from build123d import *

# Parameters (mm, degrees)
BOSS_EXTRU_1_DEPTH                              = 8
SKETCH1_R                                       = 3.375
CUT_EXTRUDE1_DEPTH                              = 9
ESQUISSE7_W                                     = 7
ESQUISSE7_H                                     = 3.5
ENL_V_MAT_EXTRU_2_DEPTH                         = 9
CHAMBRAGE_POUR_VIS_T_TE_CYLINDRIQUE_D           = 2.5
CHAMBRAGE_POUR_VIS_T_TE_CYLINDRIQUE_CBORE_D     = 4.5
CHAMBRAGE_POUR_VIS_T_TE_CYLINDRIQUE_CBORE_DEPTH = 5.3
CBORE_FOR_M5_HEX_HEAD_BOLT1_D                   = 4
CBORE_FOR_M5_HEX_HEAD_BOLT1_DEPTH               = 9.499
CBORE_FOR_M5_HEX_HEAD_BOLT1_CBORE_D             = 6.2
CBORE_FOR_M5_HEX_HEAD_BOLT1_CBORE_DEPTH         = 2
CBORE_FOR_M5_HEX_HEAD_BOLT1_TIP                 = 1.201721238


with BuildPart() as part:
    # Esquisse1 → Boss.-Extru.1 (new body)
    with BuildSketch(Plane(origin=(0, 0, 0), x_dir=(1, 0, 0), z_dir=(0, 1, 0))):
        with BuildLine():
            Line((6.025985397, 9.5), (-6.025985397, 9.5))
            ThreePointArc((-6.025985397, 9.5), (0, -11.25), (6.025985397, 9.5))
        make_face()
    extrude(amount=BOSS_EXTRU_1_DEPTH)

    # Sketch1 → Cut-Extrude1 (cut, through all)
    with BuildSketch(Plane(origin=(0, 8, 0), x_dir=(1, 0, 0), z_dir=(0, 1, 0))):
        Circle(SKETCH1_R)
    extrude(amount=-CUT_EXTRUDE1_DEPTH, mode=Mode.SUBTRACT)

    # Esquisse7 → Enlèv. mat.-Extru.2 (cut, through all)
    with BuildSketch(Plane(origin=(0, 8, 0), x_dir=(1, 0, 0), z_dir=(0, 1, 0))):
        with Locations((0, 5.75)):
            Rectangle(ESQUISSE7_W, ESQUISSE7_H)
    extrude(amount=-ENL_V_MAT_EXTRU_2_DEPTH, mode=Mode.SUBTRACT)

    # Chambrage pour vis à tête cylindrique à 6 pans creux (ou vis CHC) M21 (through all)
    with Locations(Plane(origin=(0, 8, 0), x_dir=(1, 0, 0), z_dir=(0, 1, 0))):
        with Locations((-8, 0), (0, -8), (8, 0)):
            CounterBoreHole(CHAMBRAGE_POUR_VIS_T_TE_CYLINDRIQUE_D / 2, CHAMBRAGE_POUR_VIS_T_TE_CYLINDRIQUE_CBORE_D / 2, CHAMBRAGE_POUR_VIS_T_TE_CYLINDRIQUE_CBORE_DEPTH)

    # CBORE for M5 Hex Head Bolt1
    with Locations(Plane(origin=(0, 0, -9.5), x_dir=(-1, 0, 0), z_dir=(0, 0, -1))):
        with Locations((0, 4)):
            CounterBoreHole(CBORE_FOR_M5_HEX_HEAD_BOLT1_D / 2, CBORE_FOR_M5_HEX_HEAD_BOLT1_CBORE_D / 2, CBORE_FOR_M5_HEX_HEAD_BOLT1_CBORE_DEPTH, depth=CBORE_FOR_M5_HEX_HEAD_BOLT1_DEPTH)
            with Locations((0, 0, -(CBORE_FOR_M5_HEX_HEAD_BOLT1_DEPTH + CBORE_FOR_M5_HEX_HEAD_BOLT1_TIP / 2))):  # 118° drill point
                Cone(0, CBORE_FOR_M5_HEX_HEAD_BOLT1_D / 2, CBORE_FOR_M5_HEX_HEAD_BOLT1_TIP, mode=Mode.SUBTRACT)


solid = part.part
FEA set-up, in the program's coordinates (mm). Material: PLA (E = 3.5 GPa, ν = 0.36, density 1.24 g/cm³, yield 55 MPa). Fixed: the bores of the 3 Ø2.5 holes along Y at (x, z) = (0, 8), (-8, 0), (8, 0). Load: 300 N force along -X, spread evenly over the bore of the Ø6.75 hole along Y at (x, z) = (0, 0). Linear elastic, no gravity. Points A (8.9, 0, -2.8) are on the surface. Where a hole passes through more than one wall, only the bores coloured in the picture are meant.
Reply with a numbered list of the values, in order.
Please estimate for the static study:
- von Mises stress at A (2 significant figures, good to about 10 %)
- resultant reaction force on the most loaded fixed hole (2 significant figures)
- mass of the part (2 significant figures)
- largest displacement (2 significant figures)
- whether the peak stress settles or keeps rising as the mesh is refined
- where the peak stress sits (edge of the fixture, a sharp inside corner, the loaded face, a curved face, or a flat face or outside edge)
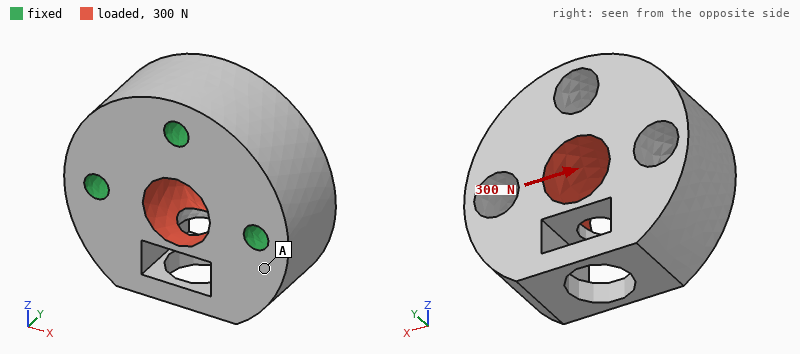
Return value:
1. 1.9 MPa
2. 130 N
3. 2.8 g
4. 21 µm
5. keeps rising
6. edge of the fixture
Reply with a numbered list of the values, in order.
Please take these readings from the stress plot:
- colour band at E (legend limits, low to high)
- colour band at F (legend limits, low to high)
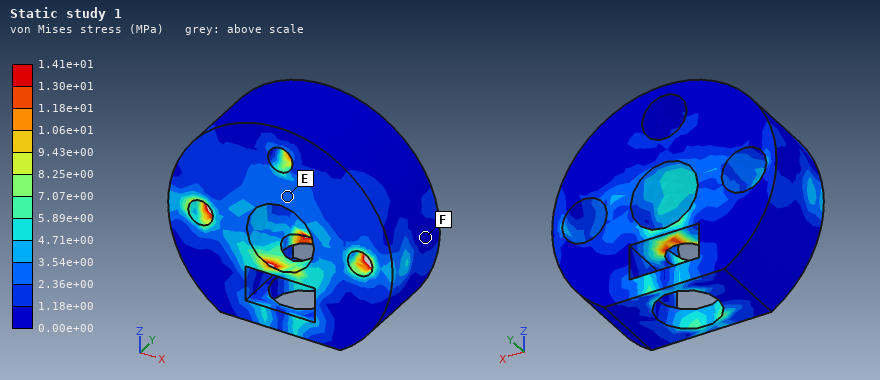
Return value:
1. 2.36e+00 to 3.54e+00 MPa
2. 0.00e+00 to 1.18e+00 MPa
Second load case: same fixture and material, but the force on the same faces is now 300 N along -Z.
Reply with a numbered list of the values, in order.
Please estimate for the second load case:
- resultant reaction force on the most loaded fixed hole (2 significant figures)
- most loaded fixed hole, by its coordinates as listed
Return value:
1. 130 N
2. (0, 8)
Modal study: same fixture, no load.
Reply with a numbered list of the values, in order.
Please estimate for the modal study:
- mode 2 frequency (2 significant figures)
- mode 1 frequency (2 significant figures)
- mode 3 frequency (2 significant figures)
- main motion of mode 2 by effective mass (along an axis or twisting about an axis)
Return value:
1. 11 kHz
2. 9200 Hz
3. 14 kHz
4. along X
